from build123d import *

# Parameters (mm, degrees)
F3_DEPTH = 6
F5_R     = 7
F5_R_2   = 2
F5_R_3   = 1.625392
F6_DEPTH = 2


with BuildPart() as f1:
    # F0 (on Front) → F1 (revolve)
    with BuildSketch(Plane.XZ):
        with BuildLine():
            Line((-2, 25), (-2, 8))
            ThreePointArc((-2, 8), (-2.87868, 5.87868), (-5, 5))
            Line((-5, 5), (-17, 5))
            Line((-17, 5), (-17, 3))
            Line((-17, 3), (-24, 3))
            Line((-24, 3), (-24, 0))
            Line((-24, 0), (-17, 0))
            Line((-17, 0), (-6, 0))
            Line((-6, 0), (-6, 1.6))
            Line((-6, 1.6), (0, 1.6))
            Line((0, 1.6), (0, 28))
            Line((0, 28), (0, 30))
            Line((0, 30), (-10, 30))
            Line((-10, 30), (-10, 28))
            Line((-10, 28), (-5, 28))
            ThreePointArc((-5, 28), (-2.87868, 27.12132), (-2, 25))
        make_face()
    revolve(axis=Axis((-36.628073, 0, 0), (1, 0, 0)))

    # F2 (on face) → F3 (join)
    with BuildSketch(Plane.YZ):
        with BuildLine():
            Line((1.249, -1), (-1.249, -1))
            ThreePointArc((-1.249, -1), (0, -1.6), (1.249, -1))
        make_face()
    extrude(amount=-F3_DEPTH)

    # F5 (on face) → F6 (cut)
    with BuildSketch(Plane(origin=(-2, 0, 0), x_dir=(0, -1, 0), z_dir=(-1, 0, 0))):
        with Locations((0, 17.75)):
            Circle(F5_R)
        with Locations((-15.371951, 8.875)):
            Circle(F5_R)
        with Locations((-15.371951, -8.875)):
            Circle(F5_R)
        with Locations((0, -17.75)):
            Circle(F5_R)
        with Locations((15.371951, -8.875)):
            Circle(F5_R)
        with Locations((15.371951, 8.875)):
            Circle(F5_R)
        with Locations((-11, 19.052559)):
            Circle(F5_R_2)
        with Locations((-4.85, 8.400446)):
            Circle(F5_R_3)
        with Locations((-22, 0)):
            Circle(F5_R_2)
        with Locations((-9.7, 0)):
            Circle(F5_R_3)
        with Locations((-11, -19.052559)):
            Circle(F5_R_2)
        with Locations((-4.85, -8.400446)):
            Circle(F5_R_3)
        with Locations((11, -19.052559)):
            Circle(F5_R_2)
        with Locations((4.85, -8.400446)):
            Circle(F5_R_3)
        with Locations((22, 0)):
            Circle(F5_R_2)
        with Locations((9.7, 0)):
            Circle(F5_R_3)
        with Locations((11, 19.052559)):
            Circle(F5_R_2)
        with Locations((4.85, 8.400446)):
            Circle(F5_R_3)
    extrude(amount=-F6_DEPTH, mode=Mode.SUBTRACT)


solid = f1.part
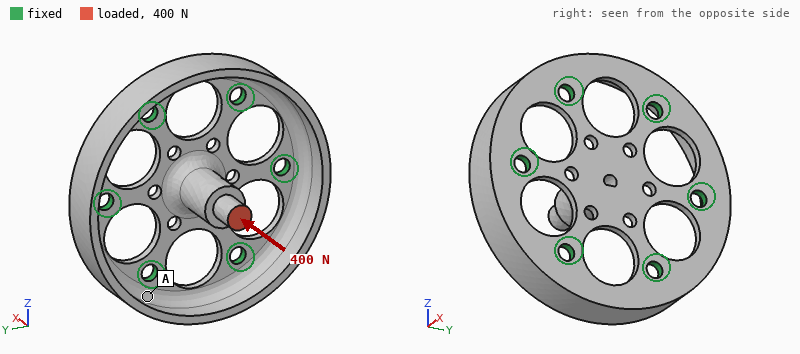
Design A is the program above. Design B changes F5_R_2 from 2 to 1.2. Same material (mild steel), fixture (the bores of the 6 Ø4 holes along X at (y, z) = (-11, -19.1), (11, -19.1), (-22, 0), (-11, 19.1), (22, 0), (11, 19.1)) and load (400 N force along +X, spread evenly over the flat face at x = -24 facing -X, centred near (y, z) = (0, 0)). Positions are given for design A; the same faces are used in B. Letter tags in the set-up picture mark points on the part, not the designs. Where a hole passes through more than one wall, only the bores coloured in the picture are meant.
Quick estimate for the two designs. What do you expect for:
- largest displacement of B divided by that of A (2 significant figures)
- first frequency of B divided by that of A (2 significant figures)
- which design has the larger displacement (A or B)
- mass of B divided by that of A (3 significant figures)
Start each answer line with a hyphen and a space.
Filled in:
- 1.2
- 0.93
- B
- 1.01
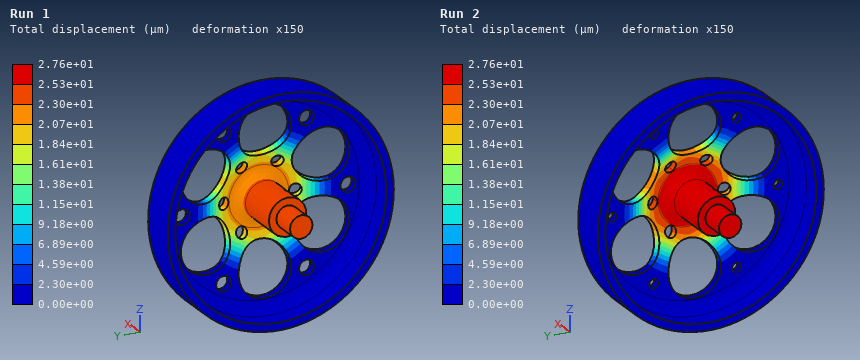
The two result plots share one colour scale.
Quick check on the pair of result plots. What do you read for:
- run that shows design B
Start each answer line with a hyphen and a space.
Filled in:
- Run 2
